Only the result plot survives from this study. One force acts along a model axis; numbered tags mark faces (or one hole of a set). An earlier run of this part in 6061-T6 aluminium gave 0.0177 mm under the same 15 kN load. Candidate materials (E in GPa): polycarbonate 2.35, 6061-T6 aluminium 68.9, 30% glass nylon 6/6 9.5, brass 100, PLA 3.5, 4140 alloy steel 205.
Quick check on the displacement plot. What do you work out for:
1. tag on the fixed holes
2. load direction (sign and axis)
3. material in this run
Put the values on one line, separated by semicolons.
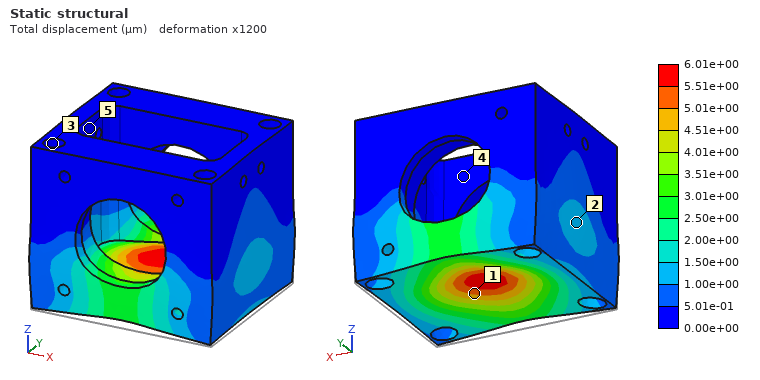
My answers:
3; +Z; 4140 alloy steel
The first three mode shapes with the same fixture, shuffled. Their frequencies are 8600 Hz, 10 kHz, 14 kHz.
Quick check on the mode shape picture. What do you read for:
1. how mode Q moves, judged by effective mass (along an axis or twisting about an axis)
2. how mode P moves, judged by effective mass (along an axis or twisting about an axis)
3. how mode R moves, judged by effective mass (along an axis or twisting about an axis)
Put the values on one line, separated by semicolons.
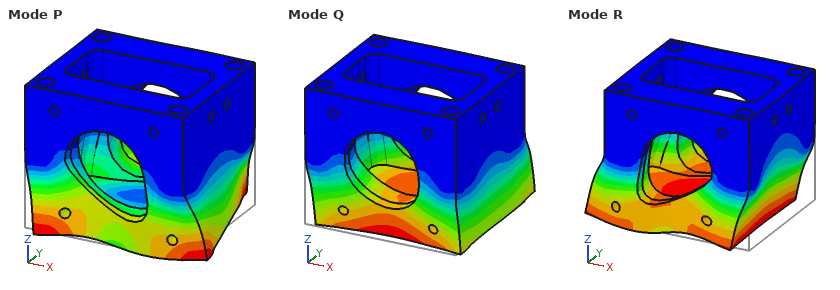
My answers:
along Y; twisting about Z; along X
